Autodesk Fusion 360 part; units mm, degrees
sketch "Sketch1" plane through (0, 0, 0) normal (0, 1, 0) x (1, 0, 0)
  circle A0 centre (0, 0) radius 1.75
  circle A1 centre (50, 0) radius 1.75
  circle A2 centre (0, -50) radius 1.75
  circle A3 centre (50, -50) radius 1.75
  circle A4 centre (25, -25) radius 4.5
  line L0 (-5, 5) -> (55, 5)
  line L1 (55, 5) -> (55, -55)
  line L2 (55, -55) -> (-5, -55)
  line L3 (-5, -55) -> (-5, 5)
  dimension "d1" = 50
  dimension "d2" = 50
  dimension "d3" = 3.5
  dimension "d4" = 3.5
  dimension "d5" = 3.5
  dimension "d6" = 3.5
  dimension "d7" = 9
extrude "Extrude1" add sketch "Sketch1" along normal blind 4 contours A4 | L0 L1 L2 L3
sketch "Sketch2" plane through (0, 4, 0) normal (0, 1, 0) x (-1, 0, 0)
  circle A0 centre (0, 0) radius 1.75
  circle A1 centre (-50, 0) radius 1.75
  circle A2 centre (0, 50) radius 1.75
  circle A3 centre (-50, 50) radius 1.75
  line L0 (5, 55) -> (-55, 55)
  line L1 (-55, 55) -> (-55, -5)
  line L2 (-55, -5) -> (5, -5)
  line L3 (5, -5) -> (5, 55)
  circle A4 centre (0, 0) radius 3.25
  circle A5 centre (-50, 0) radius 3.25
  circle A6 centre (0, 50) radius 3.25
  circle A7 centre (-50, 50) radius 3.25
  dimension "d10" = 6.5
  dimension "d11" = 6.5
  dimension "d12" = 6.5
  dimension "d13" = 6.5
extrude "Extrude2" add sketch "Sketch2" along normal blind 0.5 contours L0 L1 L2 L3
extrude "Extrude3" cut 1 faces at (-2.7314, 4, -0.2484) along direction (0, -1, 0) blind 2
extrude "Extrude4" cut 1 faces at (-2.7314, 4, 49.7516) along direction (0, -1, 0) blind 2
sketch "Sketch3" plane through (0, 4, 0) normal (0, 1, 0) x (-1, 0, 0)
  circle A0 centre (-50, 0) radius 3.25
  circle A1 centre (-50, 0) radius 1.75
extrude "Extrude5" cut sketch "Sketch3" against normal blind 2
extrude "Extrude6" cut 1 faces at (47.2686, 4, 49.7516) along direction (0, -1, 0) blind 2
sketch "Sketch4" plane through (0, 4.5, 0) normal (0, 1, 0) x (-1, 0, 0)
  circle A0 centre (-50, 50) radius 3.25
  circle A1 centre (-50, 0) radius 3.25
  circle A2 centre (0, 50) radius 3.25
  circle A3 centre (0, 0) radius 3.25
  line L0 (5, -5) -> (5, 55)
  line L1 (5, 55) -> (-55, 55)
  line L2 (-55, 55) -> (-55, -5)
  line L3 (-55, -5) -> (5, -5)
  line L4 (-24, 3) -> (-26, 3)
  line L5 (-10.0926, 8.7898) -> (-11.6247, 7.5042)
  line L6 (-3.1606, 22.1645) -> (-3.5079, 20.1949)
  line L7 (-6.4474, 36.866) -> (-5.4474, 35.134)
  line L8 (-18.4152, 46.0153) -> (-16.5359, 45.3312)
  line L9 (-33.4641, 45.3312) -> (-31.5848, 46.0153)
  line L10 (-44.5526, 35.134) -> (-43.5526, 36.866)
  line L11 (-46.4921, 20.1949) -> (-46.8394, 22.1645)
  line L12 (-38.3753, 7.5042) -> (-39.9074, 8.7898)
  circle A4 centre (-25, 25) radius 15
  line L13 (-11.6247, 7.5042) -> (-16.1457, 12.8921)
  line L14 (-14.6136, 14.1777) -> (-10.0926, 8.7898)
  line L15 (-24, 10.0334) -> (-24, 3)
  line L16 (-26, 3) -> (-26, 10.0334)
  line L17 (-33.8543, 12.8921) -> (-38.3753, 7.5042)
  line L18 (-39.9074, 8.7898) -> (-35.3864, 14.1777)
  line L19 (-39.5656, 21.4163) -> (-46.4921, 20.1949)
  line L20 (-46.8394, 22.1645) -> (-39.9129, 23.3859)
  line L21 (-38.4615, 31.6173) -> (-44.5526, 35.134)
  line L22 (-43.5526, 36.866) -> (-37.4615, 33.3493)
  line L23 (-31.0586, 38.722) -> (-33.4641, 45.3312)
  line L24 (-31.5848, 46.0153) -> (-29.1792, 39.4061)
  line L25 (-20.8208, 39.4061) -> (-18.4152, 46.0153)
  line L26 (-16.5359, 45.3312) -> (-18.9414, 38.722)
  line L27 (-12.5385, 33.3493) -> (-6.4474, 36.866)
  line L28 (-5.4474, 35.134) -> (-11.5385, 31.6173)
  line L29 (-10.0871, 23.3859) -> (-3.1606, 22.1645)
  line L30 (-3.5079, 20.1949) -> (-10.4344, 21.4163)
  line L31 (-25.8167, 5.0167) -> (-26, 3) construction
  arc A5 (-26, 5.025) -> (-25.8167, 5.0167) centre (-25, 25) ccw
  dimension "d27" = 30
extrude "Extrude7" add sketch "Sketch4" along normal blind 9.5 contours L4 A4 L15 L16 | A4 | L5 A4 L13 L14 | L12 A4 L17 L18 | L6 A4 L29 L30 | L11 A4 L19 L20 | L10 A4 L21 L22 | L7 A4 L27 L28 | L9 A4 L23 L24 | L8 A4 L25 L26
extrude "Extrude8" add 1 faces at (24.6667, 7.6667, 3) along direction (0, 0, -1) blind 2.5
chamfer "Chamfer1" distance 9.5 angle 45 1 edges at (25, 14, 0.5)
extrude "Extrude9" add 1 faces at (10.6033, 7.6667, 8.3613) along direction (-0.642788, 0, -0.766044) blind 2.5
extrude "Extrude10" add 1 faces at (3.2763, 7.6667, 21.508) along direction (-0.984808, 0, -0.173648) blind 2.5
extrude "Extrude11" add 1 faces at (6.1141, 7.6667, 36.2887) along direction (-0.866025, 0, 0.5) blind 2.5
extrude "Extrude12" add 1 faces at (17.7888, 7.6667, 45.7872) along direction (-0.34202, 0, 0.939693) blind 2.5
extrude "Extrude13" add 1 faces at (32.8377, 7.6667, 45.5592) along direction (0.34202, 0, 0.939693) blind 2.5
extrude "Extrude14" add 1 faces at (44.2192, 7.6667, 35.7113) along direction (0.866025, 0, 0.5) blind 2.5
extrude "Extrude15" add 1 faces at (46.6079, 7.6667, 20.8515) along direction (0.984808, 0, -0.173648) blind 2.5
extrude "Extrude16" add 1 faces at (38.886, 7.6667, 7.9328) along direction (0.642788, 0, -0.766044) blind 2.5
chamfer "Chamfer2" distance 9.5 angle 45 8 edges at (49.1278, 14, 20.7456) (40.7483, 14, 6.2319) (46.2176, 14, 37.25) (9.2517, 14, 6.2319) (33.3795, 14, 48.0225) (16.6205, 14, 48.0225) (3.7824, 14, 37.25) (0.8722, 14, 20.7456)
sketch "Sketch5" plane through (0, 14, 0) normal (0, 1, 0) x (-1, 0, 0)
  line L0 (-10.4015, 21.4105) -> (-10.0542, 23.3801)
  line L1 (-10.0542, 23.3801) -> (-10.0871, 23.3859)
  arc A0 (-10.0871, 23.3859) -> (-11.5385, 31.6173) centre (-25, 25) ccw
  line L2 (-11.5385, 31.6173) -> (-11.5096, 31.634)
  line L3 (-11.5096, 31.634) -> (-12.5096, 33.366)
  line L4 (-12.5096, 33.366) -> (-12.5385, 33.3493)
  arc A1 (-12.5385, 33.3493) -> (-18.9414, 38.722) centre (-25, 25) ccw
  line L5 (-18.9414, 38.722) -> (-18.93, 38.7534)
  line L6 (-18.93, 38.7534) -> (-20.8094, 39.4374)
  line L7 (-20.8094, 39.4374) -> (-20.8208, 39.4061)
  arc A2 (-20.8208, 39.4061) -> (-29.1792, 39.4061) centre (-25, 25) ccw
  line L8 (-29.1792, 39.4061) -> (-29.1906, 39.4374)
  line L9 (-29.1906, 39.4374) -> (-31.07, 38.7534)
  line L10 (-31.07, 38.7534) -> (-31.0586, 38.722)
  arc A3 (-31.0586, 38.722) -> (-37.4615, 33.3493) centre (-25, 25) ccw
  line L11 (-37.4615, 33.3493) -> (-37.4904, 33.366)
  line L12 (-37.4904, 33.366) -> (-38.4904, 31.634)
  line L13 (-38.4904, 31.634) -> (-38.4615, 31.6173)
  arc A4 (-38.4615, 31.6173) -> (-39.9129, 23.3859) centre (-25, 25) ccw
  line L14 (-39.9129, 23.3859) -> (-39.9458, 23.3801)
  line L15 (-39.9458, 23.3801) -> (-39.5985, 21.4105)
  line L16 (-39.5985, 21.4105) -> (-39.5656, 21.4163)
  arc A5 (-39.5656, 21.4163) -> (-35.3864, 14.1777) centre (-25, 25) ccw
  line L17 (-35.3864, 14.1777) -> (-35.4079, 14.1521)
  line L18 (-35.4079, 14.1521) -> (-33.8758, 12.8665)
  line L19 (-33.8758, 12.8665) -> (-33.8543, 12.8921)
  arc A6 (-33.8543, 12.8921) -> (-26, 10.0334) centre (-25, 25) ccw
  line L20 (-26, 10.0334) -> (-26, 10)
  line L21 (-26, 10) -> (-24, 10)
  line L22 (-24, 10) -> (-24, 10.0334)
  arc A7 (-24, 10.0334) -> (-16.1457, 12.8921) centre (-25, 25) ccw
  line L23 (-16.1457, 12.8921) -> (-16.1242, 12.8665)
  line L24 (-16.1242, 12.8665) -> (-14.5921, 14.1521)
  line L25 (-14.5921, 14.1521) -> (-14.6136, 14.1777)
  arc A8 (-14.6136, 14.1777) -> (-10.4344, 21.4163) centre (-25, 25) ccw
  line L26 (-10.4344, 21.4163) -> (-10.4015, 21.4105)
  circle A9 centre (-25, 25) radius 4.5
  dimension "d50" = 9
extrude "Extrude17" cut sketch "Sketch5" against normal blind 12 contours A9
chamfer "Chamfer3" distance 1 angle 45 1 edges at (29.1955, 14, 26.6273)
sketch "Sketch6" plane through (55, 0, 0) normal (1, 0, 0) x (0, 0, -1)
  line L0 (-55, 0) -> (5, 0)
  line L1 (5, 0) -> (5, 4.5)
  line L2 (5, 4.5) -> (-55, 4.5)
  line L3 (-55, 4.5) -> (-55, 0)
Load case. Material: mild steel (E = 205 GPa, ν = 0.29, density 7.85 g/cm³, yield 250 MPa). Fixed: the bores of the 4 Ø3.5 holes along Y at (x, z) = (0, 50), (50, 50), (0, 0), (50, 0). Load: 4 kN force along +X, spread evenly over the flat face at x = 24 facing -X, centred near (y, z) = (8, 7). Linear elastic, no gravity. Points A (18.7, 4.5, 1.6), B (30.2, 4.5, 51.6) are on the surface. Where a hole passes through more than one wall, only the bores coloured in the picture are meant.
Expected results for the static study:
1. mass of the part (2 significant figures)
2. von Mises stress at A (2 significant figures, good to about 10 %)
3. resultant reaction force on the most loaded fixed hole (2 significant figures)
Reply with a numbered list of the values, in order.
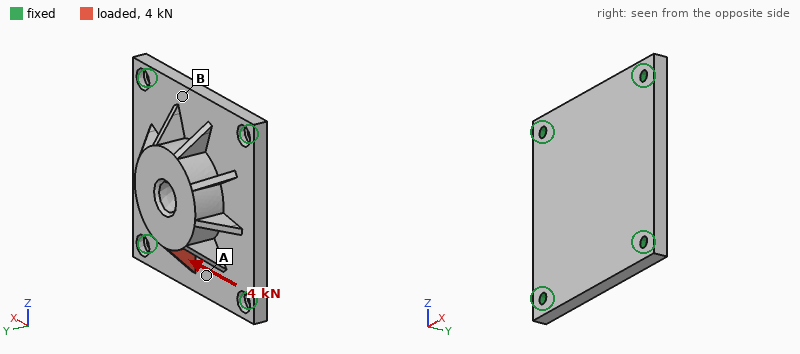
1. 180 g
2. 48 MPa
3. 1.5 kN
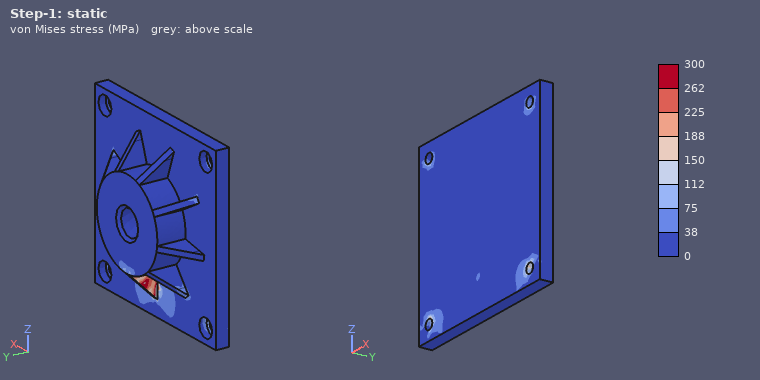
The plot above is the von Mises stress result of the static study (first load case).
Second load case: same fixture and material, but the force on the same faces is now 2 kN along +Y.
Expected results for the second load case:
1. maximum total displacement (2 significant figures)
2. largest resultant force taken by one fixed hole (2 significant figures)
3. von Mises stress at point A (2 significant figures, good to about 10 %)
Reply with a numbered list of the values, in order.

1. 32 µm
2. 1.4 kN
3. 59 MPa
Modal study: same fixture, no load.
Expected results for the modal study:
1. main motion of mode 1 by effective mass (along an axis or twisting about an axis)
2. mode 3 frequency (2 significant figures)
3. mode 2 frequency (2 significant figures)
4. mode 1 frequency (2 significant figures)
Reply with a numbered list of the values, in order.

1. along Y
2. 8400 Hz
3. 8400 Hz
4. 5100 Hz
